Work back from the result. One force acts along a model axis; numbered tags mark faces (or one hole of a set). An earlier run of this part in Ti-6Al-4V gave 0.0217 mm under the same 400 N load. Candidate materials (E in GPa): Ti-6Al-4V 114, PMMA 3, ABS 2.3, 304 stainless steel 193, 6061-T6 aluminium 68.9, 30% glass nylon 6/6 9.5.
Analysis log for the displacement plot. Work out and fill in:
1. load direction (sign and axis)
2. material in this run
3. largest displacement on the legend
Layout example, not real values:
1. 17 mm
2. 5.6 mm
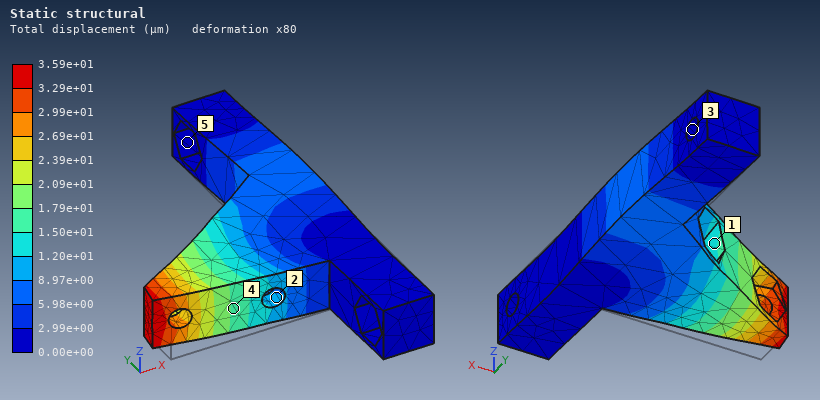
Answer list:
1. +Y
2. 6061-T6 aluminium
3. 3.59e+01 µm
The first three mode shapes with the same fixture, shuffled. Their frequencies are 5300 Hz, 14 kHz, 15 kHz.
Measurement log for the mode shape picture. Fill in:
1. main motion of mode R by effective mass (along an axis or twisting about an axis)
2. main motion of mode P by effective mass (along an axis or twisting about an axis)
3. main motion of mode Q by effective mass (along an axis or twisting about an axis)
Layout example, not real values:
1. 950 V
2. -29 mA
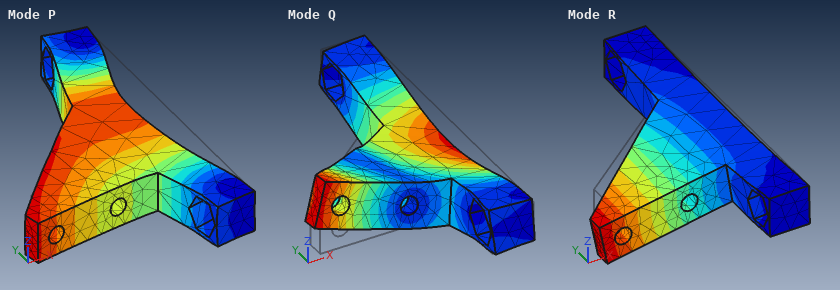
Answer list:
1. along Z
2. along X
3. along Z
